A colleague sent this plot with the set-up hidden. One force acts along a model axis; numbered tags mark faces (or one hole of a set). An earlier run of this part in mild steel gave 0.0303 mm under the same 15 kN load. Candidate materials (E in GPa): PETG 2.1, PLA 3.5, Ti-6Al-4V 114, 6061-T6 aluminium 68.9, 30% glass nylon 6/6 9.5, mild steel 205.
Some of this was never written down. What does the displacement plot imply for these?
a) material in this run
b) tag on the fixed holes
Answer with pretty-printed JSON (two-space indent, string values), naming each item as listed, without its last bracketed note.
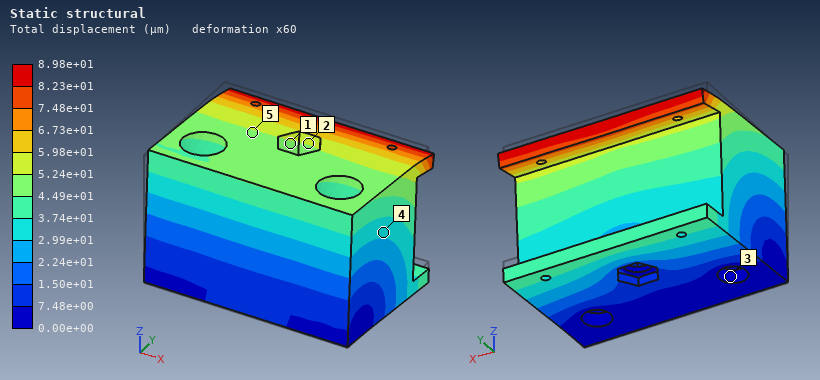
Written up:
{
  "material in this run": "6061-T6 aluminium",
  "tag on the fixed holes": "3"
}
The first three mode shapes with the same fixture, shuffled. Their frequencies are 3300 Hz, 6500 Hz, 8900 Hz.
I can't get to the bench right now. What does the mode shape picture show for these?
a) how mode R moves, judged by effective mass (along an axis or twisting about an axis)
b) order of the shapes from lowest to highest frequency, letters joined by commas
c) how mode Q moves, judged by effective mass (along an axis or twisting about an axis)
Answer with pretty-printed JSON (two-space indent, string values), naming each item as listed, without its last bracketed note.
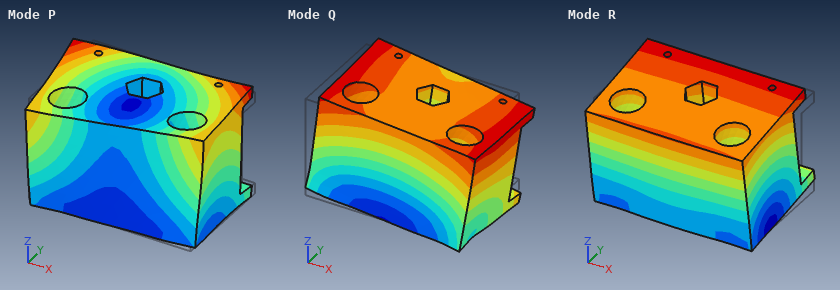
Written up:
{
  "how mode R moves, judged by effective mass": "along Y",
  "order of the shapes from lowest to highest frequency, letters joined by commas": "R, Q, P",
  "how mode Q moves, judged by effective mass": "along X"
}
